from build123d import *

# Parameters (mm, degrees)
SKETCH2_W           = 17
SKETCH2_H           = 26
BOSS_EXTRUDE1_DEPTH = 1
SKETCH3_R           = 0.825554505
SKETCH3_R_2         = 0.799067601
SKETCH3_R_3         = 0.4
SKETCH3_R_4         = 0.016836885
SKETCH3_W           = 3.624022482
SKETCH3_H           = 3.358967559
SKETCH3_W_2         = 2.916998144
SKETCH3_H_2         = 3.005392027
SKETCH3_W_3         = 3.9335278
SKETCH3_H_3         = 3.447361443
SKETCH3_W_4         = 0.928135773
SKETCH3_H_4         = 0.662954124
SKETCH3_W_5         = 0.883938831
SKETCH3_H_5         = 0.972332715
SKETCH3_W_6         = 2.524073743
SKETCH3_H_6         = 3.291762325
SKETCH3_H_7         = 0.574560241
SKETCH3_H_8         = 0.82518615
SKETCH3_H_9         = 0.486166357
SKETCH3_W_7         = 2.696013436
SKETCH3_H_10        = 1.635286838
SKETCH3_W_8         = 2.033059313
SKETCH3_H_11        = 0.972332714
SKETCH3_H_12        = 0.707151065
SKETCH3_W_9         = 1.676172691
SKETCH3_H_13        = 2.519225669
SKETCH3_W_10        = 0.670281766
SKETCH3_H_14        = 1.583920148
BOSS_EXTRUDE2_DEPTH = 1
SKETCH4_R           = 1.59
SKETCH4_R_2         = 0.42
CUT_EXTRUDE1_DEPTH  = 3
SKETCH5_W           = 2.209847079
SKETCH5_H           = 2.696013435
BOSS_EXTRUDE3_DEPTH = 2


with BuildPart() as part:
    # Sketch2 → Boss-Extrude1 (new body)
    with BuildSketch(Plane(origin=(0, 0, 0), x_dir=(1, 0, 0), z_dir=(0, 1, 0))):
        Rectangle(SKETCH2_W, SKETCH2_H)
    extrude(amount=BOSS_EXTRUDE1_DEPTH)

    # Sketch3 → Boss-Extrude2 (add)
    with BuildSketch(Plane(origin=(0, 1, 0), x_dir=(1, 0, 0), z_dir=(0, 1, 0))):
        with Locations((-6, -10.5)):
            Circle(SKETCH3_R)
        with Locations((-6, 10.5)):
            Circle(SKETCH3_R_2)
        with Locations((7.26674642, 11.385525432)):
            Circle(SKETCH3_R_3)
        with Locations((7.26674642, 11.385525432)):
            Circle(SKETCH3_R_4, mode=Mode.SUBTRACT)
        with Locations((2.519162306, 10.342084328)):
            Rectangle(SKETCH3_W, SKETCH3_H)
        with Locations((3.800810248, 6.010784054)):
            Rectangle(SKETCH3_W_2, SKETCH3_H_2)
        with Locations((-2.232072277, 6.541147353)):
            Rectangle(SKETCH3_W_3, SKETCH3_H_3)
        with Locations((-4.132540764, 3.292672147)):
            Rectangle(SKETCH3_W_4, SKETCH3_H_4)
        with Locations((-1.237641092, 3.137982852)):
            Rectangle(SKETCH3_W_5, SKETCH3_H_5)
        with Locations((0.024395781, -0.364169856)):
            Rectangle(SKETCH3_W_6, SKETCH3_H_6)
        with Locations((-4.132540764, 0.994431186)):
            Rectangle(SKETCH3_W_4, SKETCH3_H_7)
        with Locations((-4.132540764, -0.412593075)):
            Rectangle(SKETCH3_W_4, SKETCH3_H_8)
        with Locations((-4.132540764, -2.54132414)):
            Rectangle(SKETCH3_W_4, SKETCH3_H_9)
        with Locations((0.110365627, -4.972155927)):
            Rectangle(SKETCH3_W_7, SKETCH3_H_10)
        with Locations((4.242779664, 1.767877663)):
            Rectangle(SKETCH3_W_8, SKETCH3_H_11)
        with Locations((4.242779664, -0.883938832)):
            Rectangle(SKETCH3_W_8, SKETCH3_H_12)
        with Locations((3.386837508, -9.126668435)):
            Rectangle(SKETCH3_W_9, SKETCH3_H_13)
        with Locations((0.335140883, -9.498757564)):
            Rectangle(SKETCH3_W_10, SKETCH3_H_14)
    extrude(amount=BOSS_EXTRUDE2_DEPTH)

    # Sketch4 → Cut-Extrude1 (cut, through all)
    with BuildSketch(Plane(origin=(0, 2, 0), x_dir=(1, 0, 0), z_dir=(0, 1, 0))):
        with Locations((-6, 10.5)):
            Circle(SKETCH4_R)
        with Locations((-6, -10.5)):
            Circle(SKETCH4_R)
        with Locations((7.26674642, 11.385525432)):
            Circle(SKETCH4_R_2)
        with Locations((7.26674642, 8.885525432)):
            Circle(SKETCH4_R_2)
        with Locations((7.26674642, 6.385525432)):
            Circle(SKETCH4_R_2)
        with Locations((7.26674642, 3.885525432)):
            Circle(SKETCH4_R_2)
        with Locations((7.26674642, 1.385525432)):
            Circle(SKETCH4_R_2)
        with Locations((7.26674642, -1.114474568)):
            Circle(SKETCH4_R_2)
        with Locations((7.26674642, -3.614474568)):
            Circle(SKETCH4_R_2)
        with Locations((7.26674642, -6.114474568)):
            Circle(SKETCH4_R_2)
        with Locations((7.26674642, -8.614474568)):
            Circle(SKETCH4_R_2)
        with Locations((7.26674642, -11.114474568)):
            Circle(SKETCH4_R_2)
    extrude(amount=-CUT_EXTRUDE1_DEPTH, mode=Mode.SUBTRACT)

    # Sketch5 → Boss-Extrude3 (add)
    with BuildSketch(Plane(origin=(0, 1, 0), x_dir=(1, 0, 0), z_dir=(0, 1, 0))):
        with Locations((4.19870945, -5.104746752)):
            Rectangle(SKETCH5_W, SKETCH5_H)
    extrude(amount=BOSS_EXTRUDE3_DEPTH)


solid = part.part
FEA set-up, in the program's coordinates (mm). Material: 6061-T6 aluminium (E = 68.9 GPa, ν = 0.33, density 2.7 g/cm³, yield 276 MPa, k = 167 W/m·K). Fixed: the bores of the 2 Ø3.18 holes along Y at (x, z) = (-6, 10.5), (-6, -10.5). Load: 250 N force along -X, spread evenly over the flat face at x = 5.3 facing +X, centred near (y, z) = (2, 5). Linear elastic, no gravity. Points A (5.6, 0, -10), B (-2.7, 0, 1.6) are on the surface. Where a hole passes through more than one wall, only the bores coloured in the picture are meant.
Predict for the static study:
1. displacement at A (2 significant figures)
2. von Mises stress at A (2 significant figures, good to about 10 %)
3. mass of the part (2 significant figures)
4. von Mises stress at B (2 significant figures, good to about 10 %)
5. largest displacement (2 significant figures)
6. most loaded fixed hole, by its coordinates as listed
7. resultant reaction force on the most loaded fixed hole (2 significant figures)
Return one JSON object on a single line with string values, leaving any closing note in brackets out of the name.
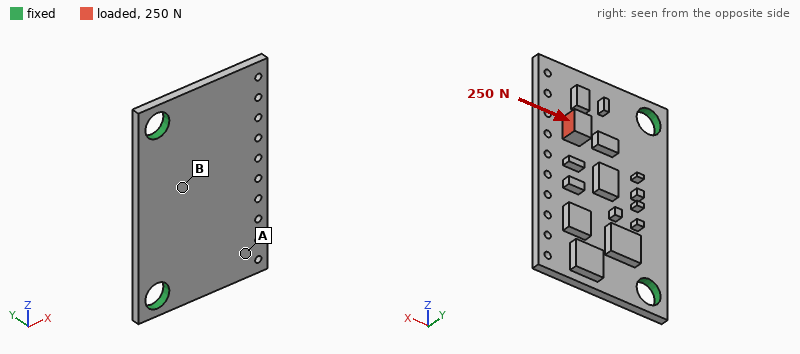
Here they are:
{"displacement at A": "0.090 mm", "von Mises stress at A": "23 MPa", "mass of the part": "1.3 g", "von Mises stress at B": "52 MPa", "largest displacement": "0.26 mm", "most loaded fixed hole, by its coordinates as listed": "(-6, 10.5)", "resultant reaction force on the most loaded fixed hole": "190 N"}
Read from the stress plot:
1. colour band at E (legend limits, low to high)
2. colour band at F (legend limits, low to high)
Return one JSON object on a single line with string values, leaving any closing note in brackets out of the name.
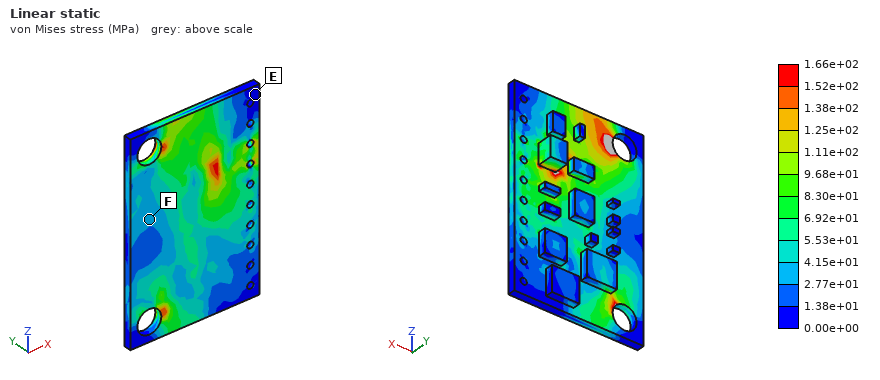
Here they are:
{"colour band at E": "0.00e+00 to 1.38e+01 MPa", "colour band at F": "2.77e+01 to 4.15e+01 MPa"}
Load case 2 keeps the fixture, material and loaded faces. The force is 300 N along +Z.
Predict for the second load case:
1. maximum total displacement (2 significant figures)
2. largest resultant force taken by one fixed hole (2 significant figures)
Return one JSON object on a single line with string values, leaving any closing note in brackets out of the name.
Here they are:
{"maximum total displacement": "0.11 mm", "largest resultant force taken by one fixed hole": "220 N"}
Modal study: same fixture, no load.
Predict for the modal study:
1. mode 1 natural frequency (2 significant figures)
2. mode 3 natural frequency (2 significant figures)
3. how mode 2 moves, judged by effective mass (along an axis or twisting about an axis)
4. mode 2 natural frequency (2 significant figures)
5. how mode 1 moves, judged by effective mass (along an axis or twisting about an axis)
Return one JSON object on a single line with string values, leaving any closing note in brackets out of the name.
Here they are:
{"mode 1 natural frequency": "3800 Hz", "mode 3 natural frequency": "12 kHz", "how mode 2 moves, judged by effective mass": "twisting about X", "mode 2 natural frequency": "7700 Hz", "how mode 1 moves, judged by effective mass": "along Y"}
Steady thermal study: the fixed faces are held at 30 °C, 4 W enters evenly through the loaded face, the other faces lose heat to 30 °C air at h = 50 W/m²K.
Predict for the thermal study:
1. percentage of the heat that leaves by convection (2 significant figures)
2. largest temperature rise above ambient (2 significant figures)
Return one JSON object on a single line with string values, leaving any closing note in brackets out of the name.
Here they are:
{"percentage of the heat that leaves by convection": "9.0 %", "largest temperature rise above ambient": "24 K"}
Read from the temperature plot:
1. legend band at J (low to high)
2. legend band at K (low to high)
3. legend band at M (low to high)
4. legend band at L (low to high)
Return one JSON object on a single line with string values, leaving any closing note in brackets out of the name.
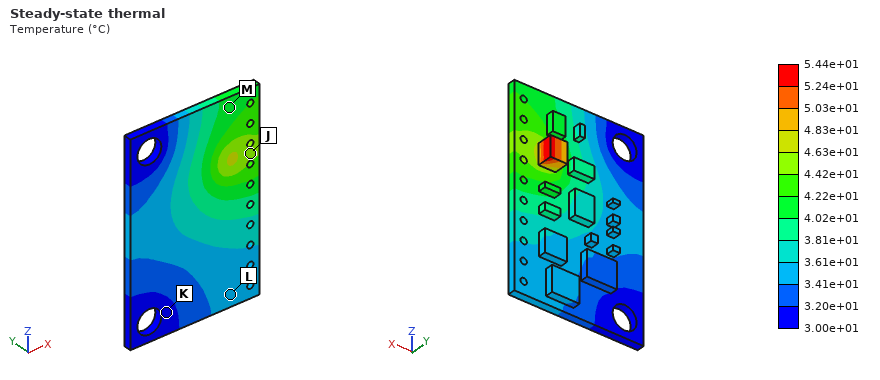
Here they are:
{"legend band at J": "4.42e+01 to 4.63e+01 °C", "legend band at K": "3.00e+01 to 3.20e+01 °C", "legend band at M": "4.02e+01 to 4.22e+01 °C", "legend band at L": "3.41e+01 to 3.61e+01 °C"}
